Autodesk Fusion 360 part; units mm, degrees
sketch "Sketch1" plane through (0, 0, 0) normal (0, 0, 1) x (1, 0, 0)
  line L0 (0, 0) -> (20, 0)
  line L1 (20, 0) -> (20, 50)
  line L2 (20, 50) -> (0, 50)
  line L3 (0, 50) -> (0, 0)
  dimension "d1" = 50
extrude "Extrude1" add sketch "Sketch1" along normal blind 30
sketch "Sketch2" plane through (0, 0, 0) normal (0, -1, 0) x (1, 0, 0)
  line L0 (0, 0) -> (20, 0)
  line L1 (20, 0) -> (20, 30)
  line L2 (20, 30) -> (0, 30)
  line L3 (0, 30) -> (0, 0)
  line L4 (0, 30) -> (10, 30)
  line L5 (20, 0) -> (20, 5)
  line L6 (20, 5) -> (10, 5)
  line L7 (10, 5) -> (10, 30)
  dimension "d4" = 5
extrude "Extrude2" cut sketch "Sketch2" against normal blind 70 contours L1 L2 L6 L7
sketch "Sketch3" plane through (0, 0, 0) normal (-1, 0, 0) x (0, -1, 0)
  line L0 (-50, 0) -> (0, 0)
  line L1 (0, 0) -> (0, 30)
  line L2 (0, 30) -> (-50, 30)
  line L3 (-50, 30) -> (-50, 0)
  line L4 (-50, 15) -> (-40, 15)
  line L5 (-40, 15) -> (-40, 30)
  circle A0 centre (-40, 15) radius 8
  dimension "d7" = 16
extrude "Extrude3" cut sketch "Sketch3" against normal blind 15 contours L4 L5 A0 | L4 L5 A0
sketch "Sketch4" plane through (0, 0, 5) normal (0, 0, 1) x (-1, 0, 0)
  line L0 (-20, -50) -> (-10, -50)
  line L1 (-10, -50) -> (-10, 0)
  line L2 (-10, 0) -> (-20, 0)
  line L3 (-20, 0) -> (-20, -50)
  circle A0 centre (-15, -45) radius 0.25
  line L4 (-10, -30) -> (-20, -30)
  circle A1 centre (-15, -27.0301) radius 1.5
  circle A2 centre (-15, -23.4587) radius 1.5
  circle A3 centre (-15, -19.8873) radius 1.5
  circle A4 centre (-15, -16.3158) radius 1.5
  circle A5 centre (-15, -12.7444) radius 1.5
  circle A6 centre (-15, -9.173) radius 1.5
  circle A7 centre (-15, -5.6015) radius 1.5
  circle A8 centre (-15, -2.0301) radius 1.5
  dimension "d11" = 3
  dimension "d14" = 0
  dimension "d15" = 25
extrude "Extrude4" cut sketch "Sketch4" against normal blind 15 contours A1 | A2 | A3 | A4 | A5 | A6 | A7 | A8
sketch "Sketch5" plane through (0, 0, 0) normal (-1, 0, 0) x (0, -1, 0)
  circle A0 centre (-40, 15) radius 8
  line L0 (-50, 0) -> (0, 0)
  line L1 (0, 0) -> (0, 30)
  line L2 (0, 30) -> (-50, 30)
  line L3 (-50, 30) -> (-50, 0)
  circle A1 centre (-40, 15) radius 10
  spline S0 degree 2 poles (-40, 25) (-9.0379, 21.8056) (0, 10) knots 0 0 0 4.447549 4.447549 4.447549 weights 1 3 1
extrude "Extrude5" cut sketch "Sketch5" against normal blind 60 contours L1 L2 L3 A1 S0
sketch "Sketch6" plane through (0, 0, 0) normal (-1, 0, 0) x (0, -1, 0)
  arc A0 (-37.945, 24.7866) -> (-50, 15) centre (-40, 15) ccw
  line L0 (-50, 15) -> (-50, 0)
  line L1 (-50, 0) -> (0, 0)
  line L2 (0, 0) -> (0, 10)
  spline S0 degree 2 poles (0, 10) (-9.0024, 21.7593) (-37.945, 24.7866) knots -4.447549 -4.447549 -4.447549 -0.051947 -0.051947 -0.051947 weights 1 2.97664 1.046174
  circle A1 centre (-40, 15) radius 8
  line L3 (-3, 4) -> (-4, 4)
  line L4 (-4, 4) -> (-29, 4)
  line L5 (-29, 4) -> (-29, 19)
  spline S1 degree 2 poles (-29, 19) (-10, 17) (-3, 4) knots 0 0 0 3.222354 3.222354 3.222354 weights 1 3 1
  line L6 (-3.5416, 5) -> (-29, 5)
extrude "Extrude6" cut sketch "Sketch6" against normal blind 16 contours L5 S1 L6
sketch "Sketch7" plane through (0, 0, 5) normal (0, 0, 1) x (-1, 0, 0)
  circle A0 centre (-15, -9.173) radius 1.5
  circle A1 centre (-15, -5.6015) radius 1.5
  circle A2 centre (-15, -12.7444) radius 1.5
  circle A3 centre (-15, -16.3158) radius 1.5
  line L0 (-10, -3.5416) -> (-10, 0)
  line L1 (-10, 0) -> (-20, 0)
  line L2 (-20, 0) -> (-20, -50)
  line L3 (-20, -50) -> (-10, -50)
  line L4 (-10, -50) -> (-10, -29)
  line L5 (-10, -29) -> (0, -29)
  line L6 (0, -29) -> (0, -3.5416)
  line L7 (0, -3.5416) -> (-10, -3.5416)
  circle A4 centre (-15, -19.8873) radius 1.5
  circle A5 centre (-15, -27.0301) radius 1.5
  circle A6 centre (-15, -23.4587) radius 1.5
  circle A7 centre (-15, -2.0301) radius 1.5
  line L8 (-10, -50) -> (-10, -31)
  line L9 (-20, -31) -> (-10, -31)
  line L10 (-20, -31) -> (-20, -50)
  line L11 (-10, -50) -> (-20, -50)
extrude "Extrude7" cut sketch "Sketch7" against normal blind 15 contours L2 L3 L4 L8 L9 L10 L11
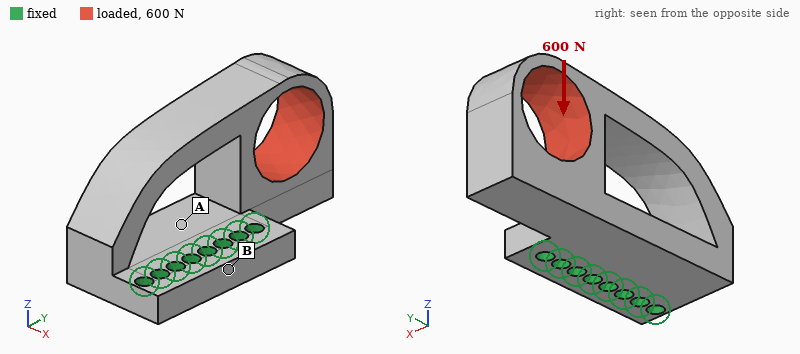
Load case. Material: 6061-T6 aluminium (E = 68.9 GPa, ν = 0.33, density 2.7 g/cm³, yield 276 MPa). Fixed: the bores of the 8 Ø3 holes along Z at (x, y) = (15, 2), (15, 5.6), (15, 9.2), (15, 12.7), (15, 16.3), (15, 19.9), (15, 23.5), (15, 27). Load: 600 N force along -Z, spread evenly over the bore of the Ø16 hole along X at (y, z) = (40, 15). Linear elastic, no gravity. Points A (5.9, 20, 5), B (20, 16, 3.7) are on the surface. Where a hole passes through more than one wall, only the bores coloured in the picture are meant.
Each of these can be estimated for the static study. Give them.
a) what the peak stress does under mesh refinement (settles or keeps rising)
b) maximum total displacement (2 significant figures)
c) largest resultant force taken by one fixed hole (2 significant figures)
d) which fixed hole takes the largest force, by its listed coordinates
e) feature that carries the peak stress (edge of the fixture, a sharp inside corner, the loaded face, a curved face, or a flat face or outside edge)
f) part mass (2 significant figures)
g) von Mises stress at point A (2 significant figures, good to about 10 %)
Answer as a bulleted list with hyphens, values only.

- keeps rising
- 0.11 mm
- 680 N
- (15, 27)
- edge of the fixture
- 20 g
- 30 MPa
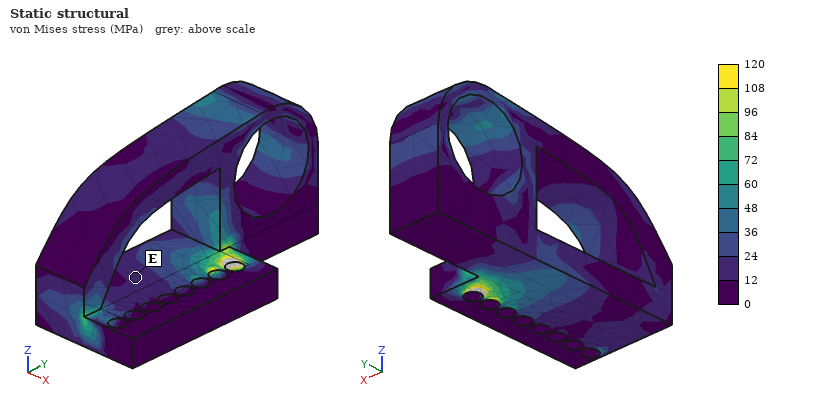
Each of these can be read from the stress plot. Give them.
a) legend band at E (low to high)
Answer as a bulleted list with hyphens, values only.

- 12 to 24 MPa
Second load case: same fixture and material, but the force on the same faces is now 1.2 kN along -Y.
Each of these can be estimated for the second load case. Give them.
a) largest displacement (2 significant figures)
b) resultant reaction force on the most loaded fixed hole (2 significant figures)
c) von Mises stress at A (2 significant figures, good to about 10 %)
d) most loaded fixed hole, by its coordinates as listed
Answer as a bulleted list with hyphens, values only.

- 0.10 mm
- 670 N
- 32 MPa
- (15, 27)
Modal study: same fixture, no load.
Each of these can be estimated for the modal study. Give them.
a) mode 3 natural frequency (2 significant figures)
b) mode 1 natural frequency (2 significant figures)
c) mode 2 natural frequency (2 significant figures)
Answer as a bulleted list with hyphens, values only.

- 8700 Hz
- 4100 Hz
- 5500 Hz
